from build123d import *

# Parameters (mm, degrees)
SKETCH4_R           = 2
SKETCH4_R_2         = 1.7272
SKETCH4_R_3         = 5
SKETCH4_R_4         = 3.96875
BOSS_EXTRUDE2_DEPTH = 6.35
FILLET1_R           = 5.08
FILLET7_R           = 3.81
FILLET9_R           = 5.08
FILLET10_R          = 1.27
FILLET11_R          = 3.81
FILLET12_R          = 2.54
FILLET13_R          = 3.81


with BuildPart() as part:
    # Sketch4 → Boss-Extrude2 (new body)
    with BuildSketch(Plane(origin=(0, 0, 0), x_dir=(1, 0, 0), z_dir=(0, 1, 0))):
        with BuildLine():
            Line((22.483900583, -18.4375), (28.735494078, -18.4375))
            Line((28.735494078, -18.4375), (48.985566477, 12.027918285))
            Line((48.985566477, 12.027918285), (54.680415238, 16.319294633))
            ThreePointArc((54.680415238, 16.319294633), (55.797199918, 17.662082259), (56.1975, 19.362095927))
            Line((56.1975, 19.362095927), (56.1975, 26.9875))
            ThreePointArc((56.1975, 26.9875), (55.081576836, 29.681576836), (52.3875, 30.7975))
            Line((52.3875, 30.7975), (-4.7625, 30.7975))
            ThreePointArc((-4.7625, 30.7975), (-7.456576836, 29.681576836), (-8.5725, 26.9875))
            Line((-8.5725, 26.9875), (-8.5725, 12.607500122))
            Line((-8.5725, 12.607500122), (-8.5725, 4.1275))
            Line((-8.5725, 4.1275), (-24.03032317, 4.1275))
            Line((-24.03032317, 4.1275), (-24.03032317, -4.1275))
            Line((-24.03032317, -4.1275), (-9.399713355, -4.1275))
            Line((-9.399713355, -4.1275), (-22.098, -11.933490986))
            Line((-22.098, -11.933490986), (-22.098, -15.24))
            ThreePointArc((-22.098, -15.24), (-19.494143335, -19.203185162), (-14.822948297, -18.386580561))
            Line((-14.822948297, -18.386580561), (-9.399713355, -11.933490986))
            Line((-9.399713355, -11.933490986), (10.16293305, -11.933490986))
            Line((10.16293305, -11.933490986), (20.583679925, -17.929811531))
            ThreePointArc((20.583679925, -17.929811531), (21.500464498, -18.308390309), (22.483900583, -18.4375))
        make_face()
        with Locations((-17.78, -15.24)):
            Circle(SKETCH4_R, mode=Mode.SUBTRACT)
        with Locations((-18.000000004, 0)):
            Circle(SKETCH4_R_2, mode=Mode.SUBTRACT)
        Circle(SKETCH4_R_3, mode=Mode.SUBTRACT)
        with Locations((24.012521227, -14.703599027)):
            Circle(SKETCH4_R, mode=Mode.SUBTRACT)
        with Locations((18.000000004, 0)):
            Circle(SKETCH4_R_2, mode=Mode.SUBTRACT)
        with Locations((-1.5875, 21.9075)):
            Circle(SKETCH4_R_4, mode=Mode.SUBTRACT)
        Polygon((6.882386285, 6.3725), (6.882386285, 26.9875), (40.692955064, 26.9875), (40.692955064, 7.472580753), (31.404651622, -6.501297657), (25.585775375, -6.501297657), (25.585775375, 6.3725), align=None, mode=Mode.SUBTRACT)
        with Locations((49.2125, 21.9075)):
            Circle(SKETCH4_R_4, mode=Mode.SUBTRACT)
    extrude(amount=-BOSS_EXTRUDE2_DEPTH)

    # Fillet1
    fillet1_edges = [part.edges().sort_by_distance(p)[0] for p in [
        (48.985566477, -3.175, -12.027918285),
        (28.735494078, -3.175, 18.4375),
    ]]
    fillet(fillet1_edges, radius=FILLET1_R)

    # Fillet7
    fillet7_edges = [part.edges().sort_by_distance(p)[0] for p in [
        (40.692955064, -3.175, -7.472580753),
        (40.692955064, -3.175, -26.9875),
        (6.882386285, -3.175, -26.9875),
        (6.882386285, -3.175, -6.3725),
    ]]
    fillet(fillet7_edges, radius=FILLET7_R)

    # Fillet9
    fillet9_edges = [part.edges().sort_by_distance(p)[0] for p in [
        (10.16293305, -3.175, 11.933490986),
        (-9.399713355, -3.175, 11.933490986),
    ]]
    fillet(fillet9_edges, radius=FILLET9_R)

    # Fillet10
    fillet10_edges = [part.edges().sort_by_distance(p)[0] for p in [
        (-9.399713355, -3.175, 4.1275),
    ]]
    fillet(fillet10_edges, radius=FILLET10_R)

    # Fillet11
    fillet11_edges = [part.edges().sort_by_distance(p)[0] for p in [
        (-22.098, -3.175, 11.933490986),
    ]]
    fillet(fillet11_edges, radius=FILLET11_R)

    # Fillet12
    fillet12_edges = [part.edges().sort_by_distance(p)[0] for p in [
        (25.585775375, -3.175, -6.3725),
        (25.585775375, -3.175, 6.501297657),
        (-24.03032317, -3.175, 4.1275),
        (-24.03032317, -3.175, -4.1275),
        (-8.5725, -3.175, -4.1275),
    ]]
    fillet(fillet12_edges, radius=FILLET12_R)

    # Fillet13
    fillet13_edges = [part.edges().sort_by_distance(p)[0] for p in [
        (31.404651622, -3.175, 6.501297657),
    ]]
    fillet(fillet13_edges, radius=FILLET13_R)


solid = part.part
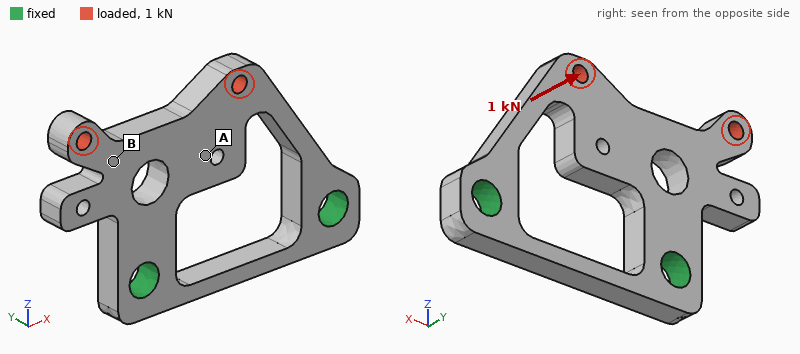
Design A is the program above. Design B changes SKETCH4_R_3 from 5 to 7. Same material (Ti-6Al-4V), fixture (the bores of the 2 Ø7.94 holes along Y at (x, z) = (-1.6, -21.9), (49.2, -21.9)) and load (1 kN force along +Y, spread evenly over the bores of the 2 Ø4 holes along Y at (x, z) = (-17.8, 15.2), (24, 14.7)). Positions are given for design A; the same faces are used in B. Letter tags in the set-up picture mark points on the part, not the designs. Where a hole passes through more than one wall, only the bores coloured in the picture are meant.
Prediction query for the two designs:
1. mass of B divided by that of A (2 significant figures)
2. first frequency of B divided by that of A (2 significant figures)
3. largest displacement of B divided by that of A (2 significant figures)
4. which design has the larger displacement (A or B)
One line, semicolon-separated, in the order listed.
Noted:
0.96; 0.95; 1.2; B
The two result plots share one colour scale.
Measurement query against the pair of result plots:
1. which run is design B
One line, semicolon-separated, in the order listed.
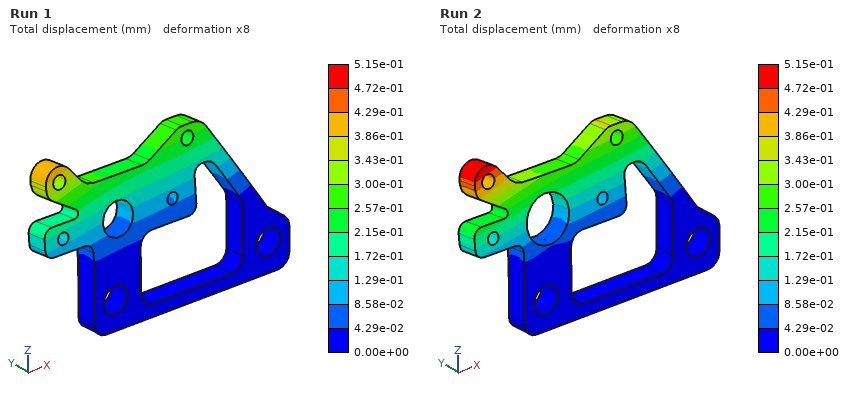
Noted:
Run 2
